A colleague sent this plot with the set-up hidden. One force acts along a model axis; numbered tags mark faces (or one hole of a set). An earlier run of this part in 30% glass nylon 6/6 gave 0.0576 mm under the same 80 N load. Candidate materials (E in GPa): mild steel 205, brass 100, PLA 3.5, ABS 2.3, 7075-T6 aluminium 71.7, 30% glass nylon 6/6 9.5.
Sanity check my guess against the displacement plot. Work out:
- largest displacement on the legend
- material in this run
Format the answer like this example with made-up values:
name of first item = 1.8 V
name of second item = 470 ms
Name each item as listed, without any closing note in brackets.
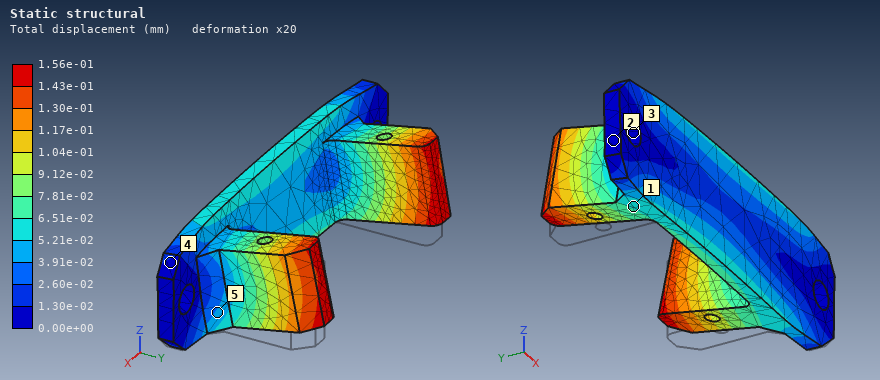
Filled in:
largest displacement on the legend = 1.56e-01 mm
material in this run = PLA
